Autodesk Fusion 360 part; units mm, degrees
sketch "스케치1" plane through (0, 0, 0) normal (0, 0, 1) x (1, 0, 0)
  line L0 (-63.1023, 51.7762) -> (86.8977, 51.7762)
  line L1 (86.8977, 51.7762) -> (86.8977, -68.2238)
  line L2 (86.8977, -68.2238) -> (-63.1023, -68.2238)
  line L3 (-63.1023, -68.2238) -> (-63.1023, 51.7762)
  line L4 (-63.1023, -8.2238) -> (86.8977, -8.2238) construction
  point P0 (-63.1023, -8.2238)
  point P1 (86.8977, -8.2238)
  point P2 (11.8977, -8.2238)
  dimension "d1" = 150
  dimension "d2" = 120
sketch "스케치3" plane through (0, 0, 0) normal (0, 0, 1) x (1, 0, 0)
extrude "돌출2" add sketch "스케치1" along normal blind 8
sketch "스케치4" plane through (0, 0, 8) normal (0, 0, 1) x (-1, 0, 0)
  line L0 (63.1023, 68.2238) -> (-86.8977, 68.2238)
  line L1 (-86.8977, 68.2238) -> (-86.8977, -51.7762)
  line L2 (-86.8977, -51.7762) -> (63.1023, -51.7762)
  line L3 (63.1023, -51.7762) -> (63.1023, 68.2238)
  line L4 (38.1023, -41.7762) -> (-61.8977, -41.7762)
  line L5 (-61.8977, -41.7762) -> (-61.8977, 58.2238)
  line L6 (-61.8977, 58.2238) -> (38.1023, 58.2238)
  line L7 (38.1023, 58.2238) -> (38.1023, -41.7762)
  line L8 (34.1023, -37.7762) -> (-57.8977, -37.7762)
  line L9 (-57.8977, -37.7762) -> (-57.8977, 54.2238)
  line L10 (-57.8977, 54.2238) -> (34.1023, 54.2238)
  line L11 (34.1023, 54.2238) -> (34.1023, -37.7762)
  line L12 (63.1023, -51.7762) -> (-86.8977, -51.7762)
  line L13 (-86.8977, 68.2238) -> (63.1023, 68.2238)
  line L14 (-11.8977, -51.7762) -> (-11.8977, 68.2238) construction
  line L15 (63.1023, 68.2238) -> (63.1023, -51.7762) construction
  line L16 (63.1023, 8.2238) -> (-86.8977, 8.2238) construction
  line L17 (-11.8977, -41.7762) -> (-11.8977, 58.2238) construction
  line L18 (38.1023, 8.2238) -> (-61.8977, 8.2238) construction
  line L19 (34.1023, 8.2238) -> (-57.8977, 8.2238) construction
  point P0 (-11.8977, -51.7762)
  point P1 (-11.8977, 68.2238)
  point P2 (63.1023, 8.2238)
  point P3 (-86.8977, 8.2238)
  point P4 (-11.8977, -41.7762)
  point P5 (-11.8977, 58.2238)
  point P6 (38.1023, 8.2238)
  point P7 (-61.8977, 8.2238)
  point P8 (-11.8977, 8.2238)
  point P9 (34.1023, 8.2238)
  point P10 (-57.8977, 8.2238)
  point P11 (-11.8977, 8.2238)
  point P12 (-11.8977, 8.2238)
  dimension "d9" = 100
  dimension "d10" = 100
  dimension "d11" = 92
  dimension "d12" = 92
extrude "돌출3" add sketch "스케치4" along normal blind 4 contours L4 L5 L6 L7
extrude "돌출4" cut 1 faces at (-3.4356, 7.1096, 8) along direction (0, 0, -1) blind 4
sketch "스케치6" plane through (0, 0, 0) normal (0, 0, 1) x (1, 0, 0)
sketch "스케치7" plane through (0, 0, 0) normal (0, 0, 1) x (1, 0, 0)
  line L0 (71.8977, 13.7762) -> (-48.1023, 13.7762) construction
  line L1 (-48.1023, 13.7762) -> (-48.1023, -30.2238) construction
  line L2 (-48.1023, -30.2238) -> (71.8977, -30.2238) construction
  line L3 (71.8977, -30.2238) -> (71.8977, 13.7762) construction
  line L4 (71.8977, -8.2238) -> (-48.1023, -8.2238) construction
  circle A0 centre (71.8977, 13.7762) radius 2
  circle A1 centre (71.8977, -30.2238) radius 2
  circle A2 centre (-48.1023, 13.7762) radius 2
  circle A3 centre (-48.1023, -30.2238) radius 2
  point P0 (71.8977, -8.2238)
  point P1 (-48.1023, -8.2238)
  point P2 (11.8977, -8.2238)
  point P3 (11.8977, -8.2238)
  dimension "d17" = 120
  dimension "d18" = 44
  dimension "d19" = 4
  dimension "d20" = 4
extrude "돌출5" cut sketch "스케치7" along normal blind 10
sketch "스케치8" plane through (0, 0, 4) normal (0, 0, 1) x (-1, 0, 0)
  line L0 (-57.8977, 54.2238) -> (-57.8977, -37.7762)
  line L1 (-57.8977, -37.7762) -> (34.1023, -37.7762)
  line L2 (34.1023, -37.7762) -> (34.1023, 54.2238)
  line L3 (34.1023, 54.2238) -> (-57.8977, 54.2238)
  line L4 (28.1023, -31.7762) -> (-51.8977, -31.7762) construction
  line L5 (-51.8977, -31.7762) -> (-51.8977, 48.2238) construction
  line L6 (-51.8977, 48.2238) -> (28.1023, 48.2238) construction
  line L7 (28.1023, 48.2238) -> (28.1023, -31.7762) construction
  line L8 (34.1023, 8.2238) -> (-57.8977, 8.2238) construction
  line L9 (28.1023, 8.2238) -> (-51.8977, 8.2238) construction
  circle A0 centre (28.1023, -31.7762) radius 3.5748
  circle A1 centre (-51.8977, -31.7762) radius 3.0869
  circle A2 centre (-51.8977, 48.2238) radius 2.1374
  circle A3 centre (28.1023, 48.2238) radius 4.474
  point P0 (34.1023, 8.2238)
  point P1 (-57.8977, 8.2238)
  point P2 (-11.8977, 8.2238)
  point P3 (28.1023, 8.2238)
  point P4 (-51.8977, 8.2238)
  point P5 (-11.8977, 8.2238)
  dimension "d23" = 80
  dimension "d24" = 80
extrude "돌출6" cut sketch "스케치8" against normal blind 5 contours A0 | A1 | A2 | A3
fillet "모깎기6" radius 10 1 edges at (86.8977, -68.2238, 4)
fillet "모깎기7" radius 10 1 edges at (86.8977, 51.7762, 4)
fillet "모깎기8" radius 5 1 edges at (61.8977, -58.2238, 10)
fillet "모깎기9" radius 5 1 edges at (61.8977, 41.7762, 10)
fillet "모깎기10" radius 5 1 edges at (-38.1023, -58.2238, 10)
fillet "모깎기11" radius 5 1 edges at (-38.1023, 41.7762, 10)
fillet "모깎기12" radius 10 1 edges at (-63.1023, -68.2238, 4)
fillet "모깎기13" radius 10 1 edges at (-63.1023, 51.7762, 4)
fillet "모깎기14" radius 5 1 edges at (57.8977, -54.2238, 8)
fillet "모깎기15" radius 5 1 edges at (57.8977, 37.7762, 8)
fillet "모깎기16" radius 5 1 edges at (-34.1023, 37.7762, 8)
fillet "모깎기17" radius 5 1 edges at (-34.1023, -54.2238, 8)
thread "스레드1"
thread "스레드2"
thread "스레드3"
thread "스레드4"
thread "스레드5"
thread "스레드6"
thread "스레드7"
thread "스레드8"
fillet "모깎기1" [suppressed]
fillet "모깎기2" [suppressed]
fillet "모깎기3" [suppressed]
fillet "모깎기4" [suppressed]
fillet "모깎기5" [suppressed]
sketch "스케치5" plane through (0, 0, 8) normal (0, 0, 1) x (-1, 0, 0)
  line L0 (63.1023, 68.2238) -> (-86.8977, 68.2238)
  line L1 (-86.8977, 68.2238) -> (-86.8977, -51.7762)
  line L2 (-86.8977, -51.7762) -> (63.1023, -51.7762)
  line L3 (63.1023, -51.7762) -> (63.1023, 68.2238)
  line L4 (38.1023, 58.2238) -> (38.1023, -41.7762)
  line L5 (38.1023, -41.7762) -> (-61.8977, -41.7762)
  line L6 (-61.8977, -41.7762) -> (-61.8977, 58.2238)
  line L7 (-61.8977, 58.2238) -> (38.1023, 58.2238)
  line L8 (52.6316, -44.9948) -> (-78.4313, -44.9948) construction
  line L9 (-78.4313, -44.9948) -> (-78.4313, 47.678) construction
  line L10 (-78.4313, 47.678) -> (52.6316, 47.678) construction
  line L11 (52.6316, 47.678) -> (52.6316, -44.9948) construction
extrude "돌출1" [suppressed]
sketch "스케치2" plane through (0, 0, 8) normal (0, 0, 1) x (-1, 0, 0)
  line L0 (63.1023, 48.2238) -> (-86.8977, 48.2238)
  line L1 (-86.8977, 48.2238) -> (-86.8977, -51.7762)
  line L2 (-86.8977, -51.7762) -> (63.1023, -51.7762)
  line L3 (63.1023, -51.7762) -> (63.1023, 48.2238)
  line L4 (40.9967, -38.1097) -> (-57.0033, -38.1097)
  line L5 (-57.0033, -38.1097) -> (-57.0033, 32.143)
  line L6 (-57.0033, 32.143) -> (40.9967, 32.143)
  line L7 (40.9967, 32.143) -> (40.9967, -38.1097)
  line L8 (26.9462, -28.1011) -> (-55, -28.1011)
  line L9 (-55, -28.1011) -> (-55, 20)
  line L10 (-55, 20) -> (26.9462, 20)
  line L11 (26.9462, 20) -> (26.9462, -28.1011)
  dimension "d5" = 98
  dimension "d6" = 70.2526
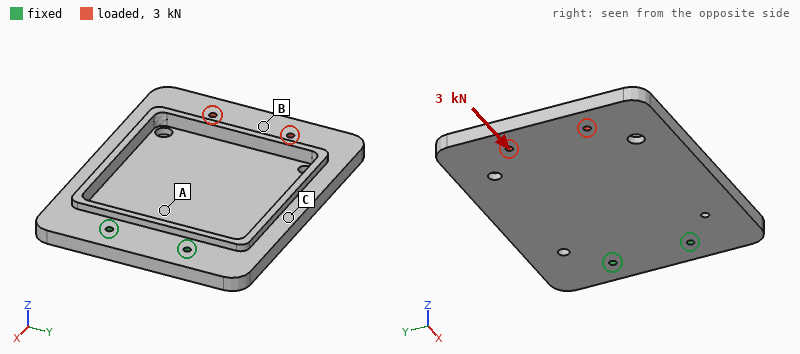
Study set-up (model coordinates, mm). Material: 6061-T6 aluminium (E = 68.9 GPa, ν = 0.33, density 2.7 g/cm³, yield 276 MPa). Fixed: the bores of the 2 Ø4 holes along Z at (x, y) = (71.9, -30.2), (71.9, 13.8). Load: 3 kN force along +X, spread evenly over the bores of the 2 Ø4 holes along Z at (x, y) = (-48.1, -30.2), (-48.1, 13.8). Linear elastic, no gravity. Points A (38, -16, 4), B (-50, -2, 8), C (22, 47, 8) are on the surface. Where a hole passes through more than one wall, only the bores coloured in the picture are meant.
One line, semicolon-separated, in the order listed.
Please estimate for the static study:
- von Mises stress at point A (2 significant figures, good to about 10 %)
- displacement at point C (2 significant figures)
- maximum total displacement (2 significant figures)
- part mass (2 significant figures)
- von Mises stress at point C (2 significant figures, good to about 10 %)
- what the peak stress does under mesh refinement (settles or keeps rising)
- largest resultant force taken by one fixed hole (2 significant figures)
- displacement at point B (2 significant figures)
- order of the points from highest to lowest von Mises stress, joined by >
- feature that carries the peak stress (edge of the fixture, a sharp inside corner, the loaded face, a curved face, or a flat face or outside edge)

11 MPa; 0.026 mm; 0.17 mm; 310 g; 7.6 MPa; keeps rising; 1.5 kN; 0.14 mm; A > C > B; edge of the fixture
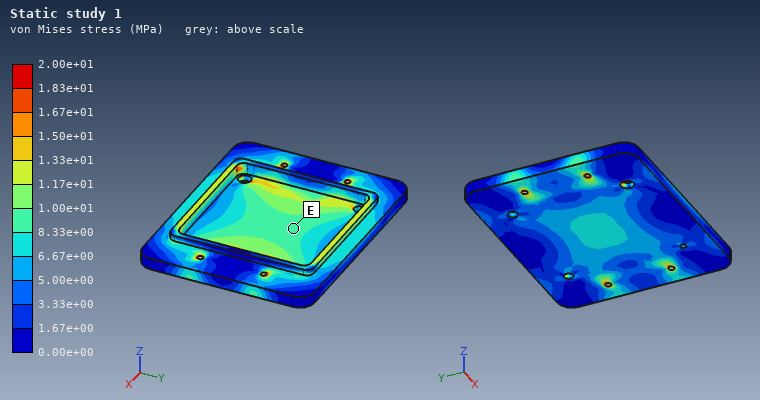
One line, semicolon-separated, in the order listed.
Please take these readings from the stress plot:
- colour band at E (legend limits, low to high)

8.33e+00 to 1.00e+01 MPa
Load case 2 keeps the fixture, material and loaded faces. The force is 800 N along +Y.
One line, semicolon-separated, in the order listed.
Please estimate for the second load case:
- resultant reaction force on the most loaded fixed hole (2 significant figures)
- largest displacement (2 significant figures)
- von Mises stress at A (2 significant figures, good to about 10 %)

2.1 kN; 76 µm; 9.0 MPa
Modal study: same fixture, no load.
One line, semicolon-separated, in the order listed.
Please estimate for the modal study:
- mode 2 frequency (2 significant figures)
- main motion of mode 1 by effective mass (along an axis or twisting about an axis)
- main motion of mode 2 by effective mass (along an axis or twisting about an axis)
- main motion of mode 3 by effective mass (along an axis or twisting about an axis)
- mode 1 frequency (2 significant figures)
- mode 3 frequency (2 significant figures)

620 Hz; along Z; twisting about X; along Z; 270 Hz; 1800 Hz
